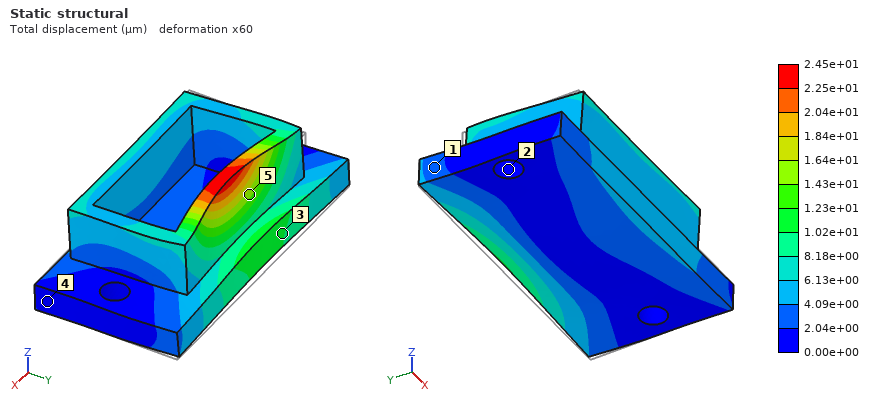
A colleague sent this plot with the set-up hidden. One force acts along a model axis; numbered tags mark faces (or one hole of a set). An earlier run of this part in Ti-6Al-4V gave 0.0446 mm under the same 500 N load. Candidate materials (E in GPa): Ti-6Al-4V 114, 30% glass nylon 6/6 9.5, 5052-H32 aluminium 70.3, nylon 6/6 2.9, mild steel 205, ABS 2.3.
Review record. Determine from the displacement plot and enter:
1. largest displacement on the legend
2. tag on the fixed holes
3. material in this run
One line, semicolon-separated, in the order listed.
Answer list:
2.45e+01 µm; 2; mild steel
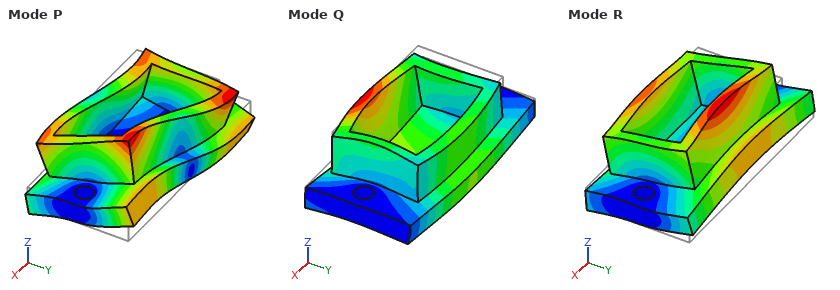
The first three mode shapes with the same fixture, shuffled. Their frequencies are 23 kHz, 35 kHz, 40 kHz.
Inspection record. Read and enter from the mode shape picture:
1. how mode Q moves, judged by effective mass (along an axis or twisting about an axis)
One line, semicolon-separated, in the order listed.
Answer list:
along Z
